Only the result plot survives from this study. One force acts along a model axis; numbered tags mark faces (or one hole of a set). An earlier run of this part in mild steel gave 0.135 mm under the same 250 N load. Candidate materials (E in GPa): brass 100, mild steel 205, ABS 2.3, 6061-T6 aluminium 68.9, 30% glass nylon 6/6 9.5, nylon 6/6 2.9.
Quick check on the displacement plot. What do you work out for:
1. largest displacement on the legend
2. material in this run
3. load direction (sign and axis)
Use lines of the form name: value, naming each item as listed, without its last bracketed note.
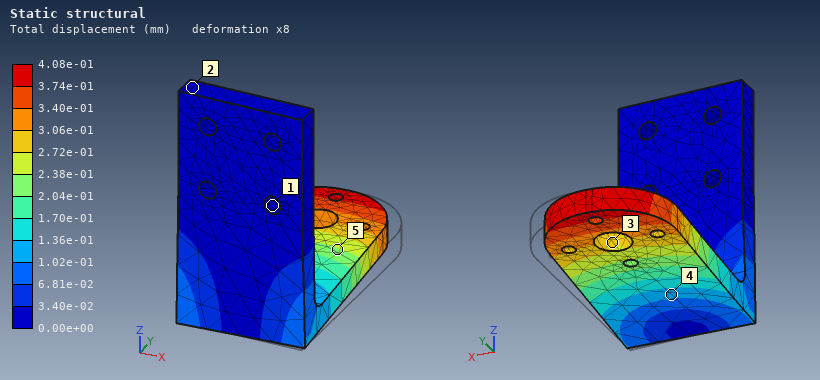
largest displacement on the legend: 4.08e-01 mm
material in this run: 6061-T6 aluminium
load direction: -X
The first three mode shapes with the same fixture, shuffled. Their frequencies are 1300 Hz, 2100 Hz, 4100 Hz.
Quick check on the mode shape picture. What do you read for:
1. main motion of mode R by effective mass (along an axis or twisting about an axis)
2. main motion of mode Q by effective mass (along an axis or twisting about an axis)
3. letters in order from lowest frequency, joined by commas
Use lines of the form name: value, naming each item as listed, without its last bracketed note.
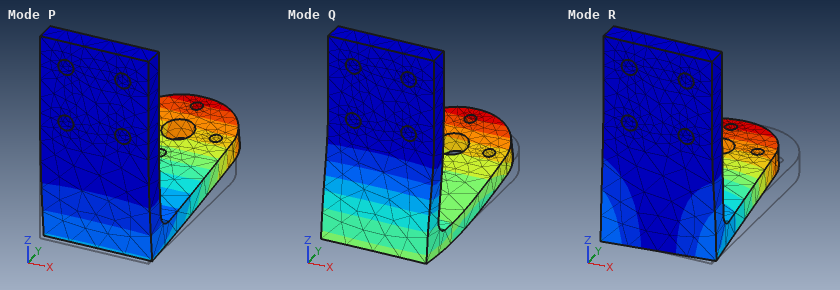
main motion of mode R by effective mass: along X
main motion of mode Q by effective mass: along Y
letters in order from lowest frequency, joined by commas: P, R, Q
